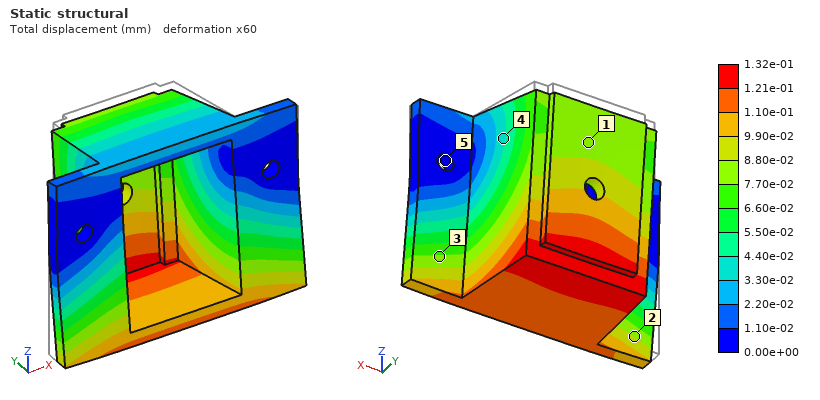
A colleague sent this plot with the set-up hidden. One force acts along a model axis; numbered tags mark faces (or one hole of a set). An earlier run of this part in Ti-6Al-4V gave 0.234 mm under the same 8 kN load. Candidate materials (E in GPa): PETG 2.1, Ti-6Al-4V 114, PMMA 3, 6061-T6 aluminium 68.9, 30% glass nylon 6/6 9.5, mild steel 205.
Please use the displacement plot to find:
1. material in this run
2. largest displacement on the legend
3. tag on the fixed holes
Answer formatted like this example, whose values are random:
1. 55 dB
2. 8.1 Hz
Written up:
1. mild steel
2. 1.32e-01 mm
3. 5
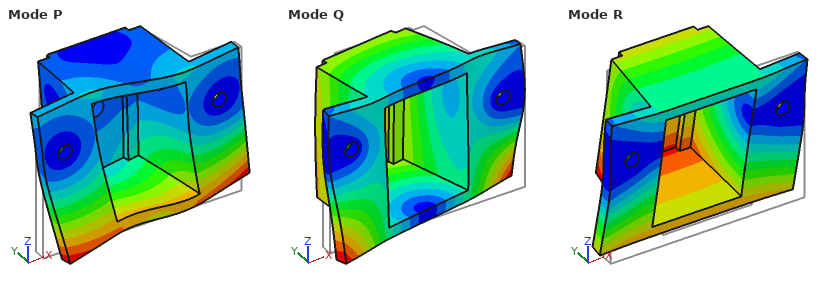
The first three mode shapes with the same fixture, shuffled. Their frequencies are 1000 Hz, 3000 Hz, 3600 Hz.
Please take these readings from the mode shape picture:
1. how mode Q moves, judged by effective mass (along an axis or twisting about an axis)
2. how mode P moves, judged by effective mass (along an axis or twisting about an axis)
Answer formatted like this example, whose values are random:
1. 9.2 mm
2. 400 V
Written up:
1. along X
2. along X
